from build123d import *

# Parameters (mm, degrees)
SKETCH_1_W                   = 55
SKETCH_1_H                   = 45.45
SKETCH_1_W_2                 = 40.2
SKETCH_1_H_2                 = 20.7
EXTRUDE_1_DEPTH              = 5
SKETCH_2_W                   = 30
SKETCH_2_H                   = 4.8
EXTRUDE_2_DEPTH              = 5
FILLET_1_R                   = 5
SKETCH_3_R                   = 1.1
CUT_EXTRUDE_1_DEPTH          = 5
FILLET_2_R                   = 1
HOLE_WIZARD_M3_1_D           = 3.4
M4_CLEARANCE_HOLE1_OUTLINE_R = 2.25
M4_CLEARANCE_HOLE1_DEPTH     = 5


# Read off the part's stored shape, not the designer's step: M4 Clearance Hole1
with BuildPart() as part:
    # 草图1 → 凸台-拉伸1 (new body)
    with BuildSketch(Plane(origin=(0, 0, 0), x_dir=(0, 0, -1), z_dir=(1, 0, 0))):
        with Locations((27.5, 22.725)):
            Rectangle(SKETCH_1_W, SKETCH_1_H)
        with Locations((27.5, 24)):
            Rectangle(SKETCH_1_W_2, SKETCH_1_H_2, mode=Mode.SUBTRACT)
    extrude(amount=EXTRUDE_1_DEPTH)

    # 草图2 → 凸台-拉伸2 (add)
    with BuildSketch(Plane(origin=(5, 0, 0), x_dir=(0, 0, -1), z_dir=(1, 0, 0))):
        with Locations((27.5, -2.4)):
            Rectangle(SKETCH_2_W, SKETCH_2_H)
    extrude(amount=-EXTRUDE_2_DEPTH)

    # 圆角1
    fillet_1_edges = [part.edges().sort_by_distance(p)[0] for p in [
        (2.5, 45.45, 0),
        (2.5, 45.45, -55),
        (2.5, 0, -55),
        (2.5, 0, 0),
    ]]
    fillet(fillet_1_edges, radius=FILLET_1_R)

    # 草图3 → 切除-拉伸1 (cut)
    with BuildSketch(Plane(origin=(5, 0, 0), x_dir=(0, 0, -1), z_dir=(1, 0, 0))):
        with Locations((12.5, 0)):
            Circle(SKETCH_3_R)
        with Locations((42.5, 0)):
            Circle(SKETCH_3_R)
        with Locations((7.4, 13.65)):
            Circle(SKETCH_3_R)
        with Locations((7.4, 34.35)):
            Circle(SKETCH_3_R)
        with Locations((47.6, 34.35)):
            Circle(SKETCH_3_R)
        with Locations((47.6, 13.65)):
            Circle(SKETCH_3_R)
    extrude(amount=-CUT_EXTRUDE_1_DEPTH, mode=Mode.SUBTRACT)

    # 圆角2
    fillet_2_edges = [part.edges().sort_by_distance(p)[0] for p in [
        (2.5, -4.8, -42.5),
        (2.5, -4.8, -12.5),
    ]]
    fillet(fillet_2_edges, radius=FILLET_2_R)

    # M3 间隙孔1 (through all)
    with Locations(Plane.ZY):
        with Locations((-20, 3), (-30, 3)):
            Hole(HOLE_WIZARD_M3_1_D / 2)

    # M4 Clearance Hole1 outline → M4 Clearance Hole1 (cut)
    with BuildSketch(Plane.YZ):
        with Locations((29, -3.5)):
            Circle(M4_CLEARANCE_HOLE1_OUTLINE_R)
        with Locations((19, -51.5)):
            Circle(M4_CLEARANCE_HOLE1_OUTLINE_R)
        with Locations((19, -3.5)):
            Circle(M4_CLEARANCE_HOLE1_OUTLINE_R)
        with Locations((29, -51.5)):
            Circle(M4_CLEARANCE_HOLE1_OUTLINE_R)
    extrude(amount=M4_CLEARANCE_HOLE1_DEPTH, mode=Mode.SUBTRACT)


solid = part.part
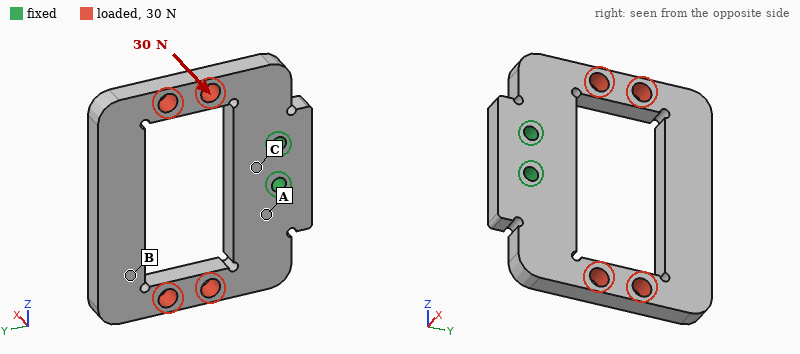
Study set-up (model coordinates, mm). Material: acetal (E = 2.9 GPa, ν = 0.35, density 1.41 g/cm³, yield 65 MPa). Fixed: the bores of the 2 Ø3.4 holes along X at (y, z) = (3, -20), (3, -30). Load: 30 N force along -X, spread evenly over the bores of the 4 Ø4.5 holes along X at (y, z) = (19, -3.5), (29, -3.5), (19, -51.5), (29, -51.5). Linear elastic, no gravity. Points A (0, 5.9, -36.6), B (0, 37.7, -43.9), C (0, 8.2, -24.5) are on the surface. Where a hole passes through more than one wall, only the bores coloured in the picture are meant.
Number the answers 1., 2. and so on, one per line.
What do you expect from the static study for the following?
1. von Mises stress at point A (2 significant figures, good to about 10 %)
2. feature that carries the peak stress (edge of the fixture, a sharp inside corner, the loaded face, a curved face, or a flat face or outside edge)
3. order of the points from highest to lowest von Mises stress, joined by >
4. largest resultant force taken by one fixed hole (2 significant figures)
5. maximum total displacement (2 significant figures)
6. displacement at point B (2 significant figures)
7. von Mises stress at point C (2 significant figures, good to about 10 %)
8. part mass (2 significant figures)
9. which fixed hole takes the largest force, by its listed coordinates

1. 4.8 MPa
2. a curved face
3. A > C > B
4. 17 N
5. 0.88 mm
6. 0.69 mm
7. 2.5 MPa
8. 12 g
9. (3, -30)
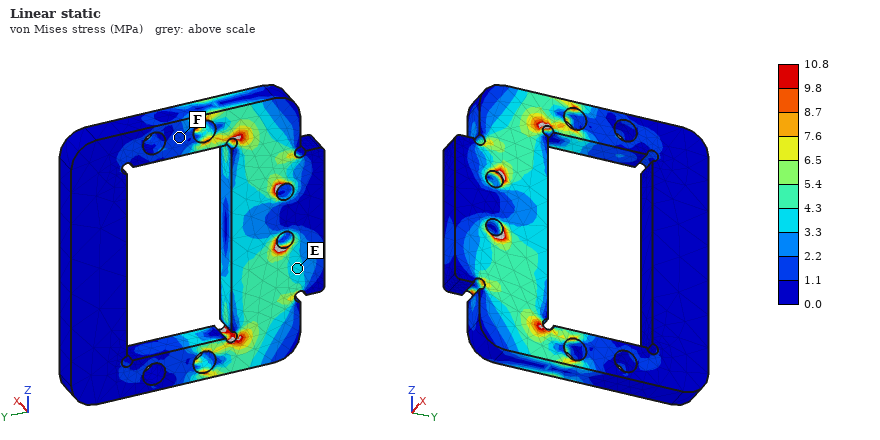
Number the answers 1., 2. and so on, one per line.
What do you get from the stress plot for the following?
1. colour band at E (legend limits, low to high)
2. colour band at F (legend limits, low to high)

1. 3.3 to 4.3 MPa
2. 1.1 to 2.2 MPa
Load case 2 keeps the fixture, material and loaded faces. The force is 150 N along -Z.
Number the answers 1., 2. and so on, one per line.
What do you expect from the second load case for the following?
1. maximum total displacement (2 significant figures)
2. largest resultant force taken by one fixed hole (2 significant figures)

1. 0.66 mm
2. 240 N
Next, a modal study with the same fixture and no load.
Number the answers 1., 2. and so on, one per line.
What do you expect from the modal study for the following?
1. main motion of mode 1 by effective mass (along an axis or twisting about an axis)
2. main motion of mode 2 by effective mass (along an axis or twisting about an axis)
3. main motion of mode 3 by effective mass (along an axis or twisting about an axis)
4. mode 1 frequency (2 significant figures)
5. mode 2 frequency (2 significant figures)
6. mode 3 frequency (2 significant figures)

1. along X
2. twisting about Y
3. along Z
4. 300 Hz
5. 690 Hz
6. 810 Hz
